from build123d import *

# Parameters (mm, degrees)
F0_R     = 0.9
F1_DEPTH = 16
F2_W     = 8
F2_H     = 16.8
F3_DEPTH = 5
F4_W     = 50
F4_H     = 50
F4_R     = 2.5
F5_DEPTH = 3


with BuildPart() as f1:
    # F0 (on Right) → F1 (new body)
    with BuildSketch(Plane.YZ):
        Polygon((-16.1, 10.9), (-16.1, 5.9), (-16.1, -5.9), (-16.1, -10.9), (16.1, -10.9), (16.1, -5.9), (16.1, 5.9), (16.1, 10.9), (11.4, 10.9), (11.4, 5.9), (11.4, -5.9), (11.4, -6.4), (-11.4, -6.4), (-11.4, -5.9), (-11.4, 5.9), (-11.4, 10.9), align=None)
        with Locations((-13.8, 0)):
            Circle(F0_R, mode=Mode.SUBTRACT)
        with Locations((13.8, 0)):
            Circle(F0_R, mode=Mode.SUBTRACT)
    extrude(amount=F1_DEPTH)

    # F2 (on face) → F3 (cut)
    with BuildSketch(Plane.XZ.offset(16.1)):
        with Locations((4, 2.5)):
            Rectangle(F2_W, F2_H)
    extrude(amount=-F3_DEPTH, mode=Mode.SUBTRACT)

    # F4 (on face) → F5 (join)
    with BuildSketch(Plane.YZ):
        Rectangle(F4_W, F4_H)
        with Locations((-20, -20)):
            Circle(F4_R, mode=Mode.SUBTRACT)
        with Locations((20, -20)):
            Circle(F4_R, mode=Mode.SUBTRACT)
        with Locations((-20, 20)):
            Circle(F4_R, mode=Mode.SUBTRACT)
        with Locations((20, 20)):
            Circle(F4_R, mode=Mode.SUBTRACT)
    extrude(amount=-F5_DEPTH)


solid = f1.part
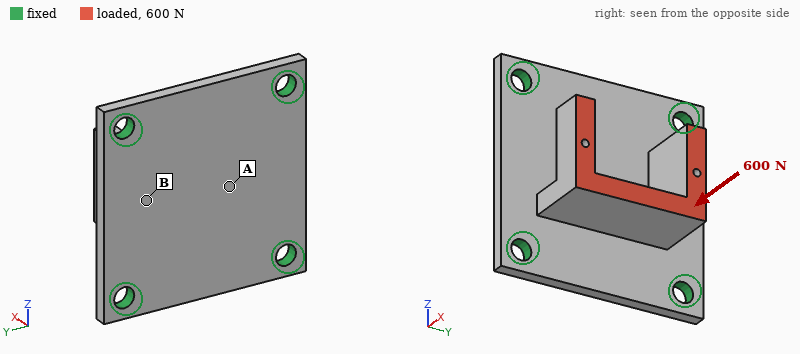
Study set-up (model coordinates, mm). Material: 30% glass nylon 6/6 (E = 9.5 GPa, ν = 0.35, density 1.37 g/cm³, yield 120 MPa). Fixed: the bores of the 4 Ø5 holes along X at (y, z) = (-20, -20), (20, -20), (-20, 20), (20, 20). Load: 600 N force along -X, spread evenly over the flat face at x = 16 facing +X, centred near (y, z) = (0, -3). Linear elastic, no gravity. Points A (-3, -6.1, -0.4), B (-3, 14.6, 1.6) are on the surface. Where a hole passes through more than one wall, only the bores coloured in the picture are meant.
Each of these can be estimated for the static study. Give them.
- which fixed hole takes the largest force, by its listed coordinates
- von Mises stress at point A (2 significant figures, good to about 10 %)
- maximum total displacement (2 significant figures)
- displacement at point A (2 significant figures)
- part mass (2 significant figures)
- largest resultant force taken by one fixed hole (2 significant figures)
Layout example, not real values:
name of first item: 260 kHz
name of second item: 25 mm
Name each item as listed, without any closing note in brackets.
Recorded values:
which fixed hole takes the largest force, by its listed coordinates: (-20, -20)
von Mises stress at point A: 15 MPa
maximum total displacement: 0.68 mm
displacement at point A: 0.15 mm
part mass: 16 g
largest resultant force taken by one fixed hole: 220 N
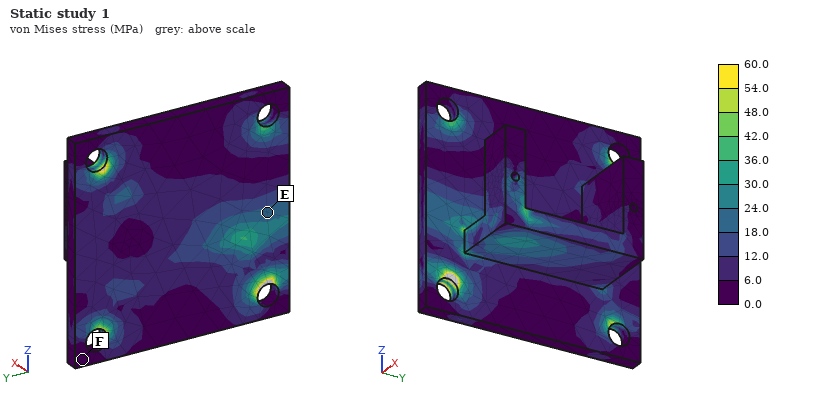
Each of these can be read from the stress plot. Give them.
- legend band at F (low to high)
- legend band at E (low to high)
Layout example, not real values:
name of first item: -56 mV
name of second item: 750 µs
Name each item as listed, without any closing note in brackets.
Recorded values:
legend band at F: 0.0 to 6.0 MPa
legend band at E: 18.0 to 24.0 MPa
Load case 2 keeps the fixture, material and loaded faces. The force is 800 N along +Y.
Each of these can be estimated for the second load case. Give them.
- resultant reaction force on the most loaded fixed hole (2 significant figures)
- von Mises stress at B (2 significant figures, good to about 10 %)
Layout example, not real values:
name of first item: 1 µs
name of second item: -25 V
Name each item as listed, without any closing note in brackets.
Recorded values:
resultant reaction force on the most loaded fixed hole: 450 N
von Mises stress at B: 6.7 MPa
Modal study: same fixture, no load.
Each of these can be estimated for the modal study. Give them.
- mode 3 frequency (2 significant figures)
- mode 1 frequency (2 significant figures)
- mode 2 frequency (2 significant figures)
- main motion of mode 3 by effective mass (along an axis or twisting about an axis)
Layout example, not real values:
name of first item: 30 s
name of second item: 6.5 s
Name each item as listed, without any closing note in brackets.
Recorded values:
mode 3 frequency: 4200 Hz
mode 1 frequency: 2600 Hz
mode 2 frequency: 3700 Hz
main motion of mode 3 by effective mass: along X
